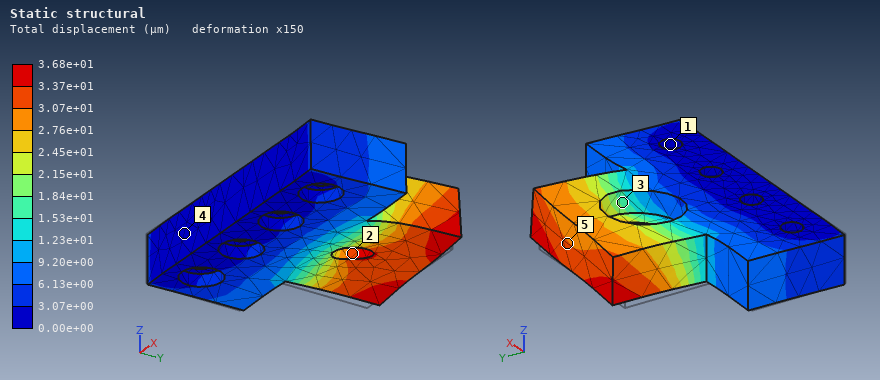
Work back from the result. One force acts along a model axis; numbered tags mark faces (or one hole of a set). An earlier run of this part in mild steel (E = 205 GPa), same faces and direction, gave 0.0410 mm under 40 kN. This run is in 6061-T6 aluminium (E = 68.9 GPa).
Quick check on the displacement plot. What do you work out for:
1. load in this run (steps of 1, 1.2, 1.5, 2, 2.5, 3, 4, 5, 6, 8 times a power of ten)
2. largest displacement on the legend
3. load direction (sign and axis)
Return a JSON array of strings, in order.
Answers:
["12 kN", "3.68e+01 µm", "+X"]
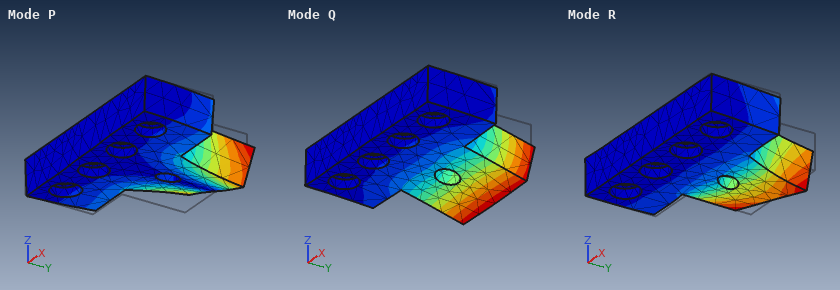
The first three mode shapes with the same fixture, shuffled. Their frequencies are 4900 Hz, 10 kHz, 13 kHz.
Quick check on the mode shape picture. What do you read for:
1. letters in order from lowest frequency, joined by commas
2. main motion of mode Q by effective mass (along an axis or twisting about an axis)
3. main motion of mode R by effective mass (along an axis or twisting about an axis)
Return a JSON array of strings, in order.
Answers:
["Q, P, R", "along Z", "along X"]
